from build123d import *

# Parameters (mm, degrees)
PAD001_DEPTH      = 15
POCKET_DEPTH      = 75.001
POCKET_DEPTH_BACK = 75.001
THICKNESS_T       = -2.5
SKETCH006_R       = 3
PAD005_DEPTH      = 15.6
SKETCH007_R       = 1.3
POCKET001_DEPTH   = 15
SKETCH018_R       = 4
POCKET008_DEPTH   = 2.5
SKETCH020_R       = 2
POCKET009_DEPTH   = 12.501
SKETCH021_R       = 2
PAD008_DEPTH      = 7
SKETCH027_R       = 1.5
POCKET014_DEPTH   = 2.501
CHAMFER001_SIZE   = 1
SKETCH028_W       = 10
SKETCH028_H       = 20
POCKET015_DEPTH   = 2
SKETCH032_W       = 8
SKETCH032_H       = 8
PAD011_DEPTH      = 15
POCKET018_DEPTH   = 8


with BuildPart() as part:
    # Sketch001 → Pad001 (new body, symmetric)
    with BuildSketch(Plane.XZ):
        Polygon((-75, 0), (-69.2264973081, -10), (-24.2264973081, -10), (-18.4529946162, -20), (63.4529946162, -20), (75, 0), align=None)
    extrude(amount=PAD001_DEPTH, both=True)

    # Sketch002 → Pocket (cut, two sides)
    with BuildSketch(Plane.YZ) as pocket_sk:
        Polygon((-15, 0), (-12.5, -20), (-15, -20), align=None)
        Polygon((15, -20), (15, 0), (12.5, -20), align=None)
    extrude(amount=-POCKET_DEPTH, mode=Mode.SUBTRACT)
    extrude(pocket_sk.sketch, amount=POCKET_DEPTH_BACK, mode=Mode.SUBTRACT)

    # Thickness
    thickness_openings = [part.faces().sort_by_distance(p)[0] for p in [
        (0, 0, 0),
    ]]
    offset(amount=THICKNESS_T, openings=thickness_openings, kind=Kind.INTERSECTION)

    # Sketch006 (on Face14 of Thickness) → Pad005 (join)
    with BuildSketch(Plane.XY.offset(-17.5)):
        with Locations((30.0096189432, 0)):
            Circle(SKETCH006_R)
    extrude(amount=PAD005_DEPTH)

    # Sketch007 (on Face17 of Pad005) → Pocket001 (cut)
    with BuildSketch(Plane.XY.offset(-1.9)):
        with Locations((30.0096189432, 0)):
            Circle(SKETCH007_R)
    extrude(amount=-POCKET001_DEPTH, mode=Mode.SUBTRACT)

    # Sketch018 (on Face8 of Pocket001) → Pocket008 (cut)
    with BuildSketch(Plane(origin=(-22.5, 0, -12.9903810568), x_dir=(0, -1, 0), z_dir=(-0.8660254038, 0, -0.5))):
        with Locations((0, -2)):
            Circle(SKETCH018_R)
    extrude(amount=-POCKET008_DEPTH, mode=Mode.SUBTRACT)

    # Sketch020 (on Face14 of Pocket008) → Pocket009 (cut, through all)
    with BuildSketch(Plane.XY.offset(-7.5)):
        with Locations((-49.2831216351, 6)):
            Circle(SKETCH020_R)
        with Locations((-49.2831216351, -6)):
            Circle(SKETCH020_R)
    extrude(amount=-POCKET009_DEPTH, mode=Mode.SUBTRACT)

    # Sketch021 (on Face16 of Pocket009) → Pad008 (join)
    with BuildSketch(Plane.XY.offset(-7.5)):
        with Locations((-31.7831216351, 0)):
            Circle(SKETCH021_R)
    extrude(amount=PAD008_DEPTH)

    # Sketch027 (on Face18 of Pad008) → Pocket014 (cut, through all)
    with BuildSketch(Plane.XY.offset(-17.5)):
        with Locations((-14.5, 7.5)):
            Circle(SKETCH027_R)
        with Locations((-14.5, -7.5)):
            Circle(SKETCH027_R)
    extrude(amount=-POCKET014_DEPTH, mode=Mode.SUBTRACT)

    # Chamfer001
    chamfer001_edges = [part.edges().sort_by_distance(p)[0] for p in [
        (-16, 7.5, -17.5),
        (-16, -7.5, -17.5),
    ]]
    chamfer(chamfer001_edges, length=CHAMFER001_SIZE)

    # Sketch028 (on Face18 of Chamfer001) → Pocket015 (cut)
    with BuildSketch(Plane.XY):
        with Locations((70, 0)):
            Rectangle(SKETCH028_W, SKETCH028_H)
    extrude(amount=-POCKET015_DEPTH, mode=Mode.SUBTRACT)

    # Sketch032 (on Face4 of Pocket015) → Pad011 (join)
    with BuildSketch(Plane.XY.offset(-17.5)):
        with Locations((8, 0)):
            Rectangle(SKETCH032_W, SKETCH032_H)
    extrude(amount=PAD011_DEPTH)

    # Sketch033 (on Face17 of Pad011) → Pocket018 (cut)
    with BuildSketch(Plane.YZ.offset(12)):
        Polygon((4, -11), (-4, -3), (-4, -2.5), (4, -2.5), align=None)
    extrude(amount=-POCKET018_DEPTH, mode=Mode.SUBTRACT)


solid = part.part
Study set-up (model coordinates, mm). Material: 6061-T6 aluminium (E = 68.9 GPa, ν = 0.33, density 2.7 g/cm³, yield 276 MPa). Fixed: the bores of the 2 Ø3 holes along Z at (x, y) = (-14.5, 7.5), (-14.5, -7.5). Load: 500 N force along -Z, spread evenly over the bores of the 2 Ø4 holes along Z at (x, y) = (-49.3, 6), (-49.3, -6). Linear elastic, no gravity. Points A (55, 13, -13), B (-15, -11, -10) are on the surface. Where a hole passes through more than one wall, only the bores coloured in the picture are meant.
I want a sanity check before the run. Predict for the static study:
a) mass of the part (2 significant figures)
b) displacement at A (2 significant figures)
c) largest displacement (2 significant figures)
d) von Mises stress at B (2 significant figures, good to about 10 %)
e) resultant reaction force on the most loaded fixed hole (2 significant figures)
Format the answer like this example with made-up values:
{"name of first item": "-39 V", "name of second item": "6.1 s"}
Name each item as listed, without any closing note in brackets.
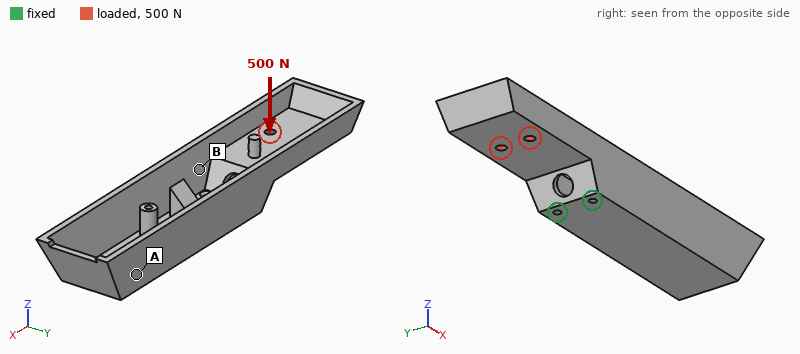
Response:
{"mass of the part": "58 g", "displacement at A": "1.2 mm", "largest displacement": "1.6 mm", "von Mises stress at B": "50 MPa", "resultant reaction force on the most loaded fixed hole": "260 N"}
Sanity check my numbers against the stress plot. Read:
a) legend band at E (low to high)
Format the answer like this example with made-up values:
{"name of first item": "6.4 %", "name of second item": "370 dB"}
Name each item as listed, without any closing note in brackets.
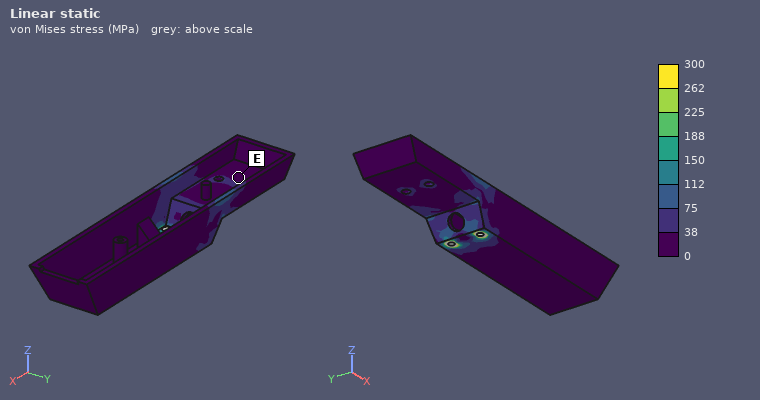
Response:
{"legend band at E": "0 to 38 MPa"}
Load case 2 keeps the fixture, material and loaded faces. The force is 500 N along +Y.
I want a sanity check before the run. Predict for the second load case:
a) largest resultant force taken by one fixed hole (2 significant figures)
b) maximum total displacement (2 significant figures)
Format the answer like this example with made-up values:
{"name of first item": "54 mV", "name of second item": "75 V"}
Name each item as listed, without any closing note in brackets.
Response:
{"largest resultant force taken by one fixed hole": "1.1 kN", "maximum total displacement": "0.15 mm"}
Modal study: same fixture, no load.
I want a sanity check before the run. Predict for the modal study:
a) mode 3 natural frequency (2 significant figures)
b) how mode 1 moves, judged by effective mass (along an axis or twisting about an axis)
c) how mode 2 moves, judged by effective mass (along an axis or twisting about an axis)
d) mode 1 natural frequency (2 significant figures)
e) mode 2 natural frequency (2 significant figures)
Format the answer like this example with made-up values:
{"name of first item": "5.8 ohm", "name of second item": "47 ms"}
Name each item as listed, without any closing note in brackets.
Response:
{"mode 3 natural frequency": "1800 Hz", "how mode 1 moves, judged by effective mass": "along Z", "how mode 2 moves, judged by effective mass": "along Y", "mode 1 natural frequency": "440 Hz", "mode 2 natural frequency": "1100 Hz"}
